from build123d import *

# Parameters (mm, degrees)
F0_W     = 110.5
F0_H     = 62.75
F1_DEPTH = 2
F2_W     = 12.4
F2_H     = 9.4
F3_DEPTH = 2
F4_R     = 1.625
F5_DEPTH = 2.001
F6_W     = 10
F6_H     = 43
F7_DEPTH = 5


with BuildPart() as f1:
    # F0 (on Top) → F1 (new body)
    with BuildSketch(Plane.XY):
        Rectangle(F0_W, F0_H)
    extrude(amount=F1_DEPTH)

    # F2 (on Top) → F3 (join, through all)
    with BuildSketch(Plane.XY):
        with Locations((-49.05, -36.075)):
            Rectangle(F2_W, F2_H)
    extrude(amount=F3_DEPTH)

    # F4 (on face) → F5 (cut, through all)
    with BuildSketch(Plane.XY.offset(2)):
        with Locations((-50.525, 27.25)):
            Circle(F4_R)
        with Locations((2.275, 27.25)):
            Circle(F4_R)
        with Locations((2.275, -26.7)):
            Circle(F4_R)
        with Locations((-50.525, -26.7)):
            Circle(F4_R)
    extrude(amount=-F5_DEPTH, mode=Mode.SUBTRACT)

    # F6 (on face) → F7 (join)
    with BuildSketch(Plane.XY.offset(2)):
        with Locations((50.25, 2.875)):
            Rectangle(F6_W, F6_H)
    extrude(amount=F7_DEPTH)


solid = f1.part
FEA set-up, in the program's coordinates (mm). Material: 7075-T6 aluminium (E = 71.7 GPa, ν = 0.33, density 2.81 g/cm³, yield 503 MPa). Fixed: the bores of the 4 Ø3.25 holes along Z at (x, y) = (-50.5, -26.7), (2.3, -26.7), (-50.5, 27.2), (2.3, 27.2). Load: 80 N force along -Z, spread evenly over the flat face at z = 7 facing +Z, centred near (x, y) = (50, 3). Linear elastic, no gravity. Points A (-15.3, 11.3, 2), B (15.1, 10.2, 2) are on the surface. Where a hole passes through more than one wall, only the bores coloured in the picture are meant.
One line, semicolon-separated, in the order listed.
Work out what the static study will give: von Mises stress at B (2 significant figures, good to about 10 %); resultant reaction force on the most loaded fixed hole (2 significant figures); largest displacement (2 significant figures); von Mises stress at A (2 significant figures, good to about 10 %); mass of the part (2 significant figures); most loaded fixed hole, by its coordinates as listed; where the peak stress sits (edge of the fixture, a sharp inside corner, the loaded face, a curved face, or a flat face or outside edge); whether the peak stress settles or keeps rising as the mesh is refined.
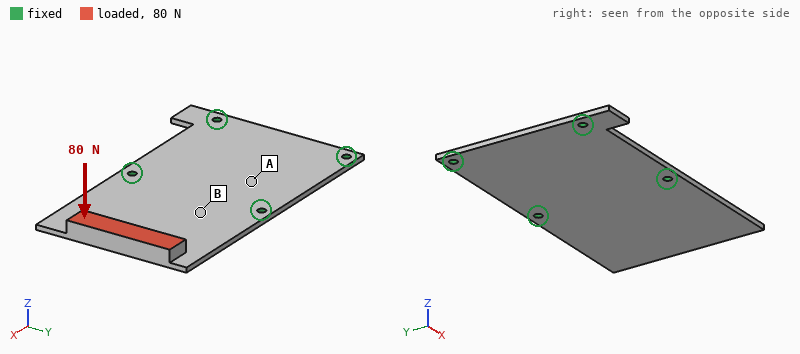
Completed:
58 MPa; 56 N; 1.3 mm; 14 MPa; 45 g; (2.3, 27.2); edge of the fixture; keeps rising
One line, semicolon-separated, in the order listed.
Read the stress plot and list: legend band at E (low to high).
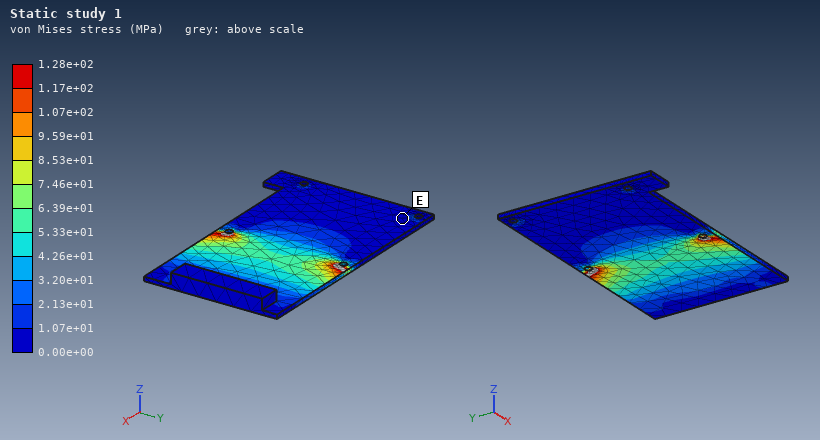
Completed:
0.00e+00 to 1.07e+01 MPa
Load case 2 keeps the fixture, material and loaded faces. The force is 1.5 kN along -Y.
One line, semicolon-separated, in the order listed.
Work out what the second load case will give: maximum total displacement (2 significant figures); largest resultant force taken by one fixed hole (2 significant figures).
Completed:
1.3 mm; 1.5 kN
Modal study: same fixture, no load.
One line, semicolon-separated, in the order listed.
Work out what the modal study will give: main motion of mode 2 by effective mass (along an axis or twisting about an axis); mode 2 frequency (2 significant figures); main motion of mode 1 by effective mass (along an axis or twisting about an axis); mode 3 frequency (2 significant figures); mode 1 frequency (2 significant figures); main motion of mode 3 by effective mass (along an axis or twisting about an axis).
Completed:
twisting about X; 1200 Hz; along Z; 2500 Hz; 380 Hz; along Z
